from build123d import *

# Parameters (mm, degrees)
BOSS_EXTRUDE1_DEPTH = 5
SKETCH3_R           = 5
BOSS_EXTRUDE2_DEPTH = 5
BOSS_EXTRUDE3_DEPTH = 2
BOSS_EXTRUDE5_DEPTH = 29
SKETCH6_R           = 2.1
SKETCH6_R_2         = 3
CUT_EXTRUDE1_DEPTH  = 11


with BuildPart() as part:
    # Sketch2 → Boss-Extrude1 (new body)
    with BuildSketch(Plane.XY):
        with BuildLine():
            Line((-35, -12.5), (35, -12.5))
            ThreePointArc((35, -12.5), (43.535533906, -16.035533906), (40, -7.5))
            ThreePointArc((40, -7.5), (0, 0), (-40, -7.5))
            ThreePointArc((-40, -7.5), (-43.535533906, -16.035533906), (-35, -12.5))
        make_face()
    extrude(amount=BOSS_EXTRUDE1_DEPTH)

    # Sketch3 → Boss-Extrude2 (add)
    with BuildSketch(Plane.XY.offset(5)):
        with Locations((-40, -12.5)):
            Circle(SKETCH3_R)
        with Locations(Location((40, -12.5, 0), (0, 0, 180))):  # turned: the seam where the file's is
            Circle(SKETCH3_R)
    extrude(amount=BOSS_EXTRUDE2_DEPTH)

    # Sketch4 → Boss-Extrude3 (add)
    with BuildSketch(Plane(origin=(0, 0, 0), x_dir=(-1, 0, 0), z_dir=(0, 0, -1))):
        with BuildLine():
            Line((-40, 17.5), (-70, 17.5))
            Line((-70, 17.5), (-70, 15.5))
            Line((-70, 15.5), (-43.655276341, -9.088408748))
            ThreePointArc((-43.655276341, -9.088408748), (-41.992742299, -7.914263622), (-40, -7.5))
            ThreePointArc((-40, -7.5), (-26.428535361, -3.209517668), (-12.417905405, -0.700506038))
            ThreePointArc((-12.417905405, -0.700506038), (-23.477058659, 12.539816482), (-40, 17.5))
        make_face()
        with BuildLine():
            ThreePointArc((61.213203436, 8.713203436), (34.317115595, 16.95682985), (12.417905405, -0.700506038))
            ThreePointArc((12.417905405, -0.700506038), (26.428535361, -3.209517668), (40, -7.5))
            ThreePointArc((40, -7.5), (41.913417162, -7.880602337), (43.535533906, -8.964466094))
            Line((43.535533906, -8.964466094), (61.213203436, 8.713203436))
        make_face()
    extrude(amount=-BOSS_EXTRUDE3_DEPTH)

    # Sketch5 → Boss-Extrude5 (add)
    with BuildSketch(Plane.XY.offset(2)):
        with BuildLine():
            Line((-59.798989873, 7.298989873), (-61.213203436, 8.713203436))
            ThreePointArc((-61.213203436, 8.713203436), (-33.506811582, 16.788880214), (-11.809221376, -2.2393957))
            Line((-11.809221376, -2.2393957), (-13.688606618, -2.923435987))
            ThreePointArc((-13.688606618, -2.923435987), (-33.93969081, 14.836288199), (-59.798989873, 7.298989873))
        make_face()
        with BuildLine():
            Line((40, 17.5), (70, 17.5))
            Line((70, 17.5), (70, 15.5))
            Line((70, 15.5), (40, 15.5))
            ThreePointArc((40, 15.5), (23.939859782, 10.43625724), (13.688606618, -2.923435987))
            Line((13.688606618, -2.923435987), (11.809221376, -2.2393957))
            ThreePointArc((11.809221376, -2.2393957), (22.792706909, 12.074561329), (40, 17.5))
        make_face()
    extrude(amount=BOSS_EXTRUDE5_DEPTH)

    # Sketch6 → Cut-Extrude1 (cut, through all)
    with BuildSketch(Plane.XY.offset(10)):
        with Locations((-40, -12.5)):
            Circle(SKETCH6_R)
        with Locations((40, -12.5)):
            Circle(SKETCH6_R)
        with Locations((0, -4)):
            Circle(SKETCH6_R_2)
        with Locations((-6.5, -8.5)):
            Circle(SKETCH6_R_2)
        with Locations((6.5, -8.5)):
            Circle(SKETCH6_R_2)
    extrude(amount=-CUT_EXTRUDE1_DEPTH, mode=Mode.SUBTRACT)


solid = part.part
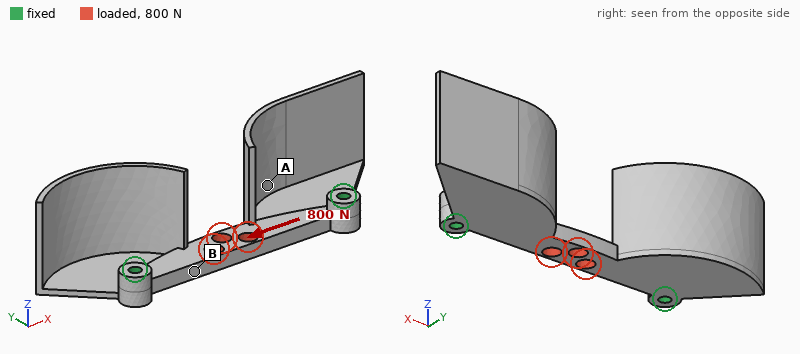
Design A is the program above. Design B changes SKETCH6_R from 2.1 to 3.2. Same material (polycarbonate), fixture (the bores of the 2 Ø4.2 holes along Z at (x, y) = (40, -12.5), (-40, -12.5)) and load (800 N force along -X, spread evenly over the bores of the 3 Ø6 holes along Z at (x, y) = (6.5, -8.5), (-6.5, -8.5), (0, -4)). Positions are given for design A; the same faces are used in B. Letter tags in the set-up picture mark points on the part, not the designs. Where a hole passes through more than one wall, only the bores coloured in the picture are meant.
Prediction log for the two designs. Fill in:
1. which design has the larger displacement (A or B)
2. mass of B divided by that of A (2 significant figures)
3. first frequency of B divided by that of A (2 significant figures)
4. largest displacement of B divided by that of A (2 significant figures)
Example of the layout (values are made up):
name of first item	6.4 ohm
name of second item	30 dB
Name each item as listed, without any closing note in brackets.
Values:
which design has the larger displacement	A
mass of B divided by that of A	0.98
first frequency of B divided by that of A	1.0
largest displacement of B divided by that of A	0.90
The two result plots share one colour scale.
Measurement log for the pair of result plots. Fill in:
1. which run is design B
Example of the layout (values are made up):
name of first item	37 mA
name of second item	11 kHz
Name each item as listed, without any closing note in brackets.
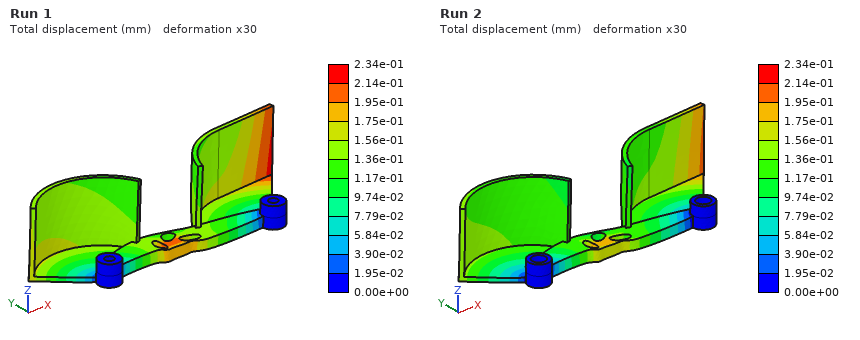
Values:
which run is design B	Run 2
